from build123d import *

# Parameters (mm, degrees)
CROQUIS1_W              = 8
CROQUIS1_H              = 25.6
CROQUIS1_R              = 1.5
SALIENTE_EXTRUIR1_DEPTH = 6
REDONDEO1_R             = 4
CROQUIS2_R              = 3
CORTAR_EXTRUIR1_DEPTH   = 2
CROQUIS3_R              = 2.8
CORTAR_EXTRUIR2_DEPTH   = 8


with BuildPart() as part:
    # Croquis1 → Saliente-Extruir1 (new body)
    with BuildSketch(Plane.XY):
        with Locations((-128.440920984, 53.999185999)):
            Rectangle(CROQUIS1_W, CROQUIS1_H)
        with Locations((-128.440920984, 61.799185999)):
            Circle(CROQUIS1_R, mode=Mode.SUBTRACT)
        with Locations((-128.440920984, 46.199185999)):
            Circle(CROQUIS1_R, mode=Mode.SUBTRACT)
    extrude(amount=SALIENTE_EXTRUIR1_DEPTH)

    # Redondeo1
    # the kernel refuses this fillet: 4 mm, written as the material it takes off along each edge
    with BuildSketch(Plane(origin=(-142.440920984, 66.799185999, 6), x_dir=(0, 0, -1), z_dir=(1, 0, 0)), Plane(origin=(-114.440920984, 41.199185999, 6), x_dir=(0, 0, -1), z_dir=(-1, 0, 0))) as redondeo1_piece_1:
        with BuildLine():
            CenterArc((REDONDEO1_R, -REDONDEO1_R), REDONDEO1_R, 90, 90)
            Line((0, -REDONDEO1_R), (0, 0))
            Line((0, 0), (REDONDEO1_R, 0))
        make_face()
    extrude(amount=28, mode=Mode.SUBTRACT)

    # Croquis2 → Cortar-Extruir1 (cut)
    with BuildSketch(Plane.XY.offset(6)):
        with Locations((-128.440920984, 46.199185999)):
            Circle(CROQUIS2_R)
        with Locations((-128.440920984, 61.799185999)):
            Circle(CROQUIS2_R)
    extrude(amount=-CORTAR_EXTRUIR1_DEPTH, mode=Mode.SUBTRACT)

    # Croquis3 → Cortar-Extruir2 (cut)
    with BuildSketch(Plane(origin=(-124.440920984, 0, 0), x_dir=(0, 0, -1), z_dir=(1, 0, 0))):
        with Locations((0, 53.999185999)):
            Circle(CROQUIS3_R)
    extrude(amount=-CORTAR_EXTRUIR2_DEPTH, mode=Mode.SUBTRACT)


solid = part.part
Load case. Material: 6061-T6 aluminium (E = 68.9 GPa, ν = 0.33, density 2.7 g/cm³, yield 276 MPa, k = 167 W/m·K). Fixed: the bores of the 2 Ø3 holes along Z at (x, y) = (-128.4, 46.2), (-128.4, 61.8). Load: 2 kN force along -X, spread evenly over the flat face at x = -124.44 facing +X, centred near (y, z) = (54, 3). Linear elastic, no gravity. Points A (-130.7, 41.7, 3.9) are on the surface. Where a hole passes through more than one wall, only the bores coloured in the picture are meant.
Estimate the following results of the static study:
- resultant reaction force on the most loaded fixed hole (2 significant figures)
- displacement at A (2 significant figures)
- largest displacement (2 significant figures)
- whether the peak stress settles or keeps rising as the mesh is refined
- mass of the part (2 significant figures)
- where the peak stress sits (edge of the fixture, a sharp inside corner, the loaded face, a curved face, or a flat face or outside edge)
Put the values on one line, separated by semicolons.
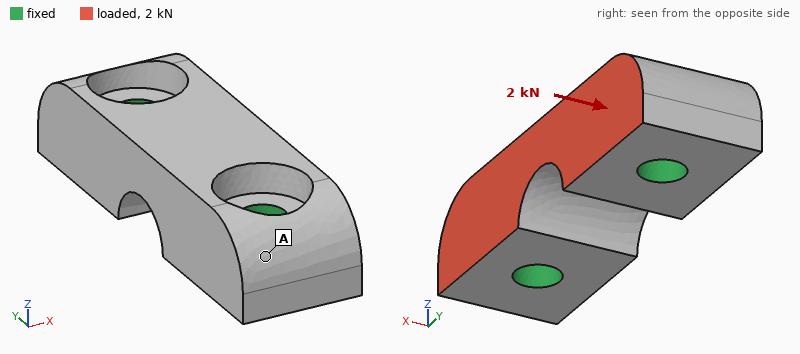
1.0 kN; 1.1 µm; 7.5 µm; keeps rising; 2.5 g; edge of the fixture
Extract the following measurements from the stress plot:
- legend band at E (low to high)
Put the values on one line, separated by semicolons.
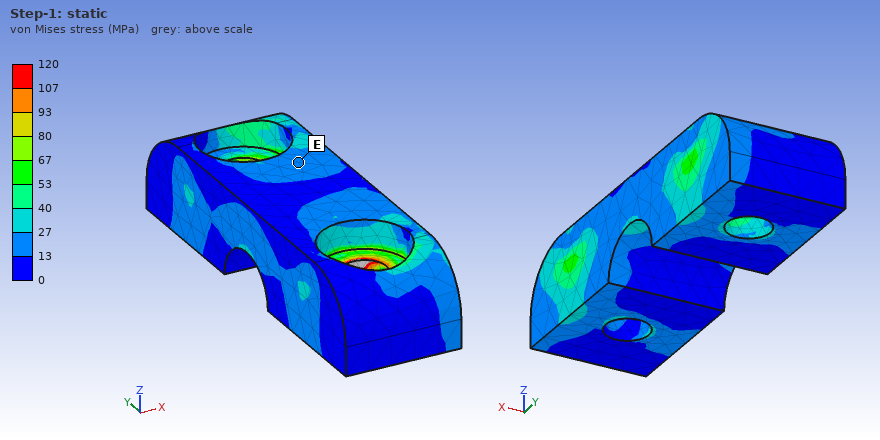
13 to 27 MPa
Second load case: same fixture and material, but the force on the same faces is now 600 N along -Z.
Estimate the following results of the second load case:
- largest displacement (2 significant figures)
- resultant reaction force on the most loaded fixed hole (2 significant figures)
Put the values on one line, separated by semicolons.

5.0 µm; 310 N
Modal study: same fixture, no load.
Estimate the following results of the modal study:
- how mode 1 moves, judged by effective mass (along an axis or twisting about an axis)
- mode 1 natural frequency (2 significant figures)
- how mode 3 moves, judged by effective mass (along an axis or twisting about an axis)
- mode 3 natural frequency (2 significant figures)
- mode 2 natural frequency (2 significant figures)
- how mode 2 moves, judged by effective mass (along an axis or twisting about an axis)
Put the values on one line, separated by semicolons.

along X; 60 kHz; twisting about Y; 92 kHz; 75 kHz; along Z
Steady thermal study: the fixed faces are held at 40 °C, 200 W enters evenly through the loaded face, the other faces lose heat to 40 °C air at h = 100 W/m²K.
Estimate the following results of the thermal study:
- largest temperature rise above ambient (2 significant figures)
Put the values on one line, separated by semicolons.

64 K
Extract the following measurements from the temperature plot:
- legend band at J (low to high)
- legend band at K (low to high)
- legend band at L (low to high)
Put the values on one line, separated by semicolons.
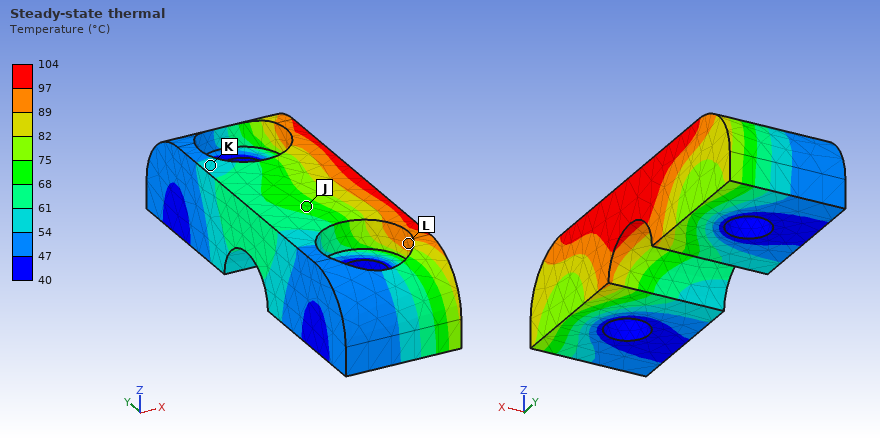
68 to 75 °C; 54 to 61 °C; 89 to 97 °C
